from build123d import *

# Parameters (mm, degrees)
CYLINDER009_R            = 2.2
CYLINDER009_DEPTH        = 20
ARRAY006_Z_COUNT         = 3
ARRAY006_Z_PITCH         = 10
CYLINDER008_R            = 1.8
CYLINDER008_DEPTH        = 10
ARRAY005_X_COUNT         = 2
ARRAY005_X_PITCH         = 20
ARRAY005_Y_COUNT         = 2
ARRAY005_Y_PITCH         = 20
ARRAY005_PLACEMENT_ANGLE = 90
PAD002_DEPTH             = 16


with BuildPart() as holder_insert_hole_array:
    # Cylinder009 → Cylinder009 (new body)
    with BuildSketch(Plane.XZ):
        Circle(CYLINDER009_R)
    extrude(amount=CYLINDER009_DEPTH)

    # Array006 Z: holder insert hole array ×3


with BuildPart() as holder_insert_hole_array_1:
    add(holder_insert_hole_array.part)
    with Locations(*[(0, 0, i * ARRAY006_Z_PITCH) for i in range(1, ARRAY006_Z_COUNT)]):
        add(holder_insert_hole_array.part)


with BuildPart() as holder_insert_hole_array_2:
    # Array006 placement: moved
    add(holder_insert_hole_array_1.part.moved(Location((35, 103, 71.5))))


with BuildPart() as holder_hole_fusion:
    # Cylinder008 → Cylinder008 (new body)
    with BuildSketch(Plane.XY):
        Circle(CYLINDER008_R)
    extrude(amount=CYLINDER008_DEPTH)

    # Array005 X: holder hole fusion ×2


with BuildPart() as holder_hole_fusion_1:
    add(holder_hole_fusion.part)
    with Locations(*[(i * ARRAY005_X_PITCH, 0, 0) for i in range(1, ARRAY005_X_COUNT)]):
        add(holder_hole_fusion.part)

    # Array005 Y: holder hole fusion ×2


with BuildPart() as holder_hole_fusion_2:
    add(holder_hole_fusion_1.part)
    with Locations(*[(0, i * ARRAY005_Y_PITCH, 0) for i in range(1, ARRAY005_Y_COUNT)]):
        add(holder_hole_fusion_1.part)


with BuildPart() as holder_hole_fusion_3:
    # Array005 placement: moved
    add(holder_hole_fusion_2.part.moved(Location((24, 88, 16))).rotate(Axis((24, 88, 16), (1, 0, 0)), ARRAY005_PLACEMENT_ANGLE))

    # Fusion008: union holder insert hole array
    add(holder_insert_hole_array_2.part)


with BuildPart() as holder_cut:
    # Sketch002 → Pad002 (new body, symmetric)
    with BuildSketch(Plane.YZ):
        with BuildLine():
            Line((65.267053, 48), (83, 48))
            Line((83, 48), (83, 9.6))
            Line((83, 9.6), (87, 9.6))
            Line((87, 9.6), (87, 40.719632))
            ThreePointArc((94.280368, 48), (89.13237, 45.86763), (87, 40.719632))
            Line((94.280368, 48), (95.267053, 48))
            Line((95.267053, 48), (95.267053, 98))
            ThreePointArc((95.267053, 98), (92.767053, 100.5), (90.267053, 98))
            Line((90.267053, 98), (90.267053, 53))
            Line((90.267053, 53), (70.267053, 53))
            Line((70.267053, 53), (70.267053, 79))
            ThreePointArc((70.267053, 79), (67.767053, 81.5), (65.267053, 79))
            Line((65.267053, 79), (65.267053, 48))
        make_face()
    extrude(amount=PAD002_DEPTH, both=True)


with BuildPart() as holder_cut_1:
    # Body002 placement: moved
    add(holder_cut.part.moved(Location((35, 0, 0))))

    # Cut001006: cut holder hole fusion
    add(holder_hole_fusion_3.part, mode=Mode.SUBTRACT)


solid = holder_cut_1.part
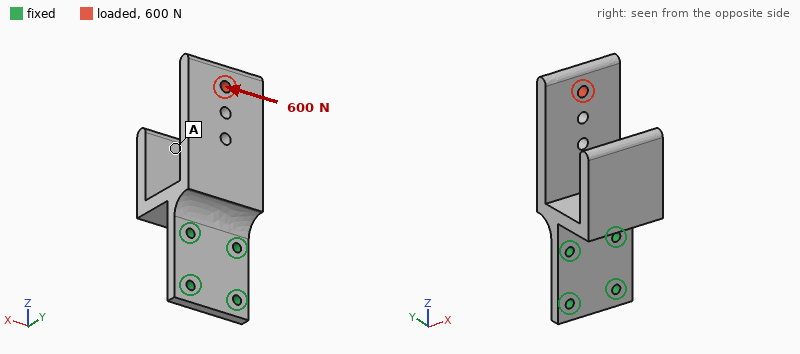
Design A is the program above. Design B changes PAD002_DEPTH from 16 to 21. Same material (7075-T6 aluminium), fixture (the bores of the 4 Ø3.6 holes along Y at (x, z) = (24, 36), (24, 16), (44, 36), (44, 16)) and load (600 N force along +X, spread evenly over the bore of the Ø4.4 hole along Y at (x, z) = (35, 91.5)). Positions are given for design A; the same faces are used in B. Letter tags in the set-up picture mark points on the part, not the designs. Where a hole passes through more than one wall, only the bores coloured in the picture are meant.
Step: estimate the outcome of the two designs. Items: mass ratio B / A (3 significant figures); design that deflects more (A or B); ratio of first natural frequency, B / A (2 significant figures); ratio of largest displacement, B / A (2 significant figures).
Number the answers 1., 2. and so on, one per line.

1. 1.32
2. A
3. 0.98
4. 0.65
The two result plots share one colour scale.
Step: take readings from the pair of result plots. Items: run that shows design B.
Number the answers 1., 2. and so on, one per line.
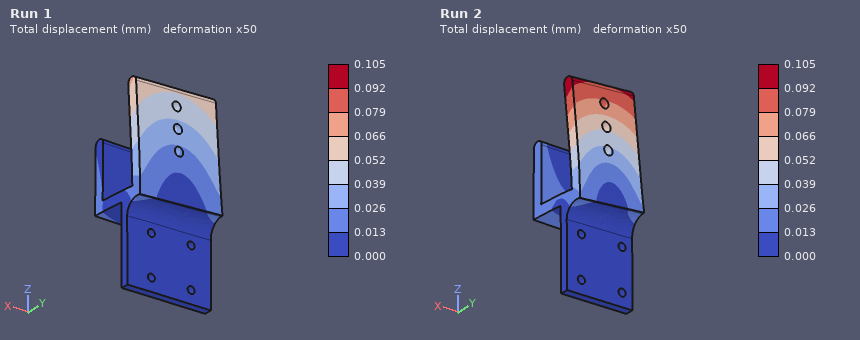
1. Run 1
